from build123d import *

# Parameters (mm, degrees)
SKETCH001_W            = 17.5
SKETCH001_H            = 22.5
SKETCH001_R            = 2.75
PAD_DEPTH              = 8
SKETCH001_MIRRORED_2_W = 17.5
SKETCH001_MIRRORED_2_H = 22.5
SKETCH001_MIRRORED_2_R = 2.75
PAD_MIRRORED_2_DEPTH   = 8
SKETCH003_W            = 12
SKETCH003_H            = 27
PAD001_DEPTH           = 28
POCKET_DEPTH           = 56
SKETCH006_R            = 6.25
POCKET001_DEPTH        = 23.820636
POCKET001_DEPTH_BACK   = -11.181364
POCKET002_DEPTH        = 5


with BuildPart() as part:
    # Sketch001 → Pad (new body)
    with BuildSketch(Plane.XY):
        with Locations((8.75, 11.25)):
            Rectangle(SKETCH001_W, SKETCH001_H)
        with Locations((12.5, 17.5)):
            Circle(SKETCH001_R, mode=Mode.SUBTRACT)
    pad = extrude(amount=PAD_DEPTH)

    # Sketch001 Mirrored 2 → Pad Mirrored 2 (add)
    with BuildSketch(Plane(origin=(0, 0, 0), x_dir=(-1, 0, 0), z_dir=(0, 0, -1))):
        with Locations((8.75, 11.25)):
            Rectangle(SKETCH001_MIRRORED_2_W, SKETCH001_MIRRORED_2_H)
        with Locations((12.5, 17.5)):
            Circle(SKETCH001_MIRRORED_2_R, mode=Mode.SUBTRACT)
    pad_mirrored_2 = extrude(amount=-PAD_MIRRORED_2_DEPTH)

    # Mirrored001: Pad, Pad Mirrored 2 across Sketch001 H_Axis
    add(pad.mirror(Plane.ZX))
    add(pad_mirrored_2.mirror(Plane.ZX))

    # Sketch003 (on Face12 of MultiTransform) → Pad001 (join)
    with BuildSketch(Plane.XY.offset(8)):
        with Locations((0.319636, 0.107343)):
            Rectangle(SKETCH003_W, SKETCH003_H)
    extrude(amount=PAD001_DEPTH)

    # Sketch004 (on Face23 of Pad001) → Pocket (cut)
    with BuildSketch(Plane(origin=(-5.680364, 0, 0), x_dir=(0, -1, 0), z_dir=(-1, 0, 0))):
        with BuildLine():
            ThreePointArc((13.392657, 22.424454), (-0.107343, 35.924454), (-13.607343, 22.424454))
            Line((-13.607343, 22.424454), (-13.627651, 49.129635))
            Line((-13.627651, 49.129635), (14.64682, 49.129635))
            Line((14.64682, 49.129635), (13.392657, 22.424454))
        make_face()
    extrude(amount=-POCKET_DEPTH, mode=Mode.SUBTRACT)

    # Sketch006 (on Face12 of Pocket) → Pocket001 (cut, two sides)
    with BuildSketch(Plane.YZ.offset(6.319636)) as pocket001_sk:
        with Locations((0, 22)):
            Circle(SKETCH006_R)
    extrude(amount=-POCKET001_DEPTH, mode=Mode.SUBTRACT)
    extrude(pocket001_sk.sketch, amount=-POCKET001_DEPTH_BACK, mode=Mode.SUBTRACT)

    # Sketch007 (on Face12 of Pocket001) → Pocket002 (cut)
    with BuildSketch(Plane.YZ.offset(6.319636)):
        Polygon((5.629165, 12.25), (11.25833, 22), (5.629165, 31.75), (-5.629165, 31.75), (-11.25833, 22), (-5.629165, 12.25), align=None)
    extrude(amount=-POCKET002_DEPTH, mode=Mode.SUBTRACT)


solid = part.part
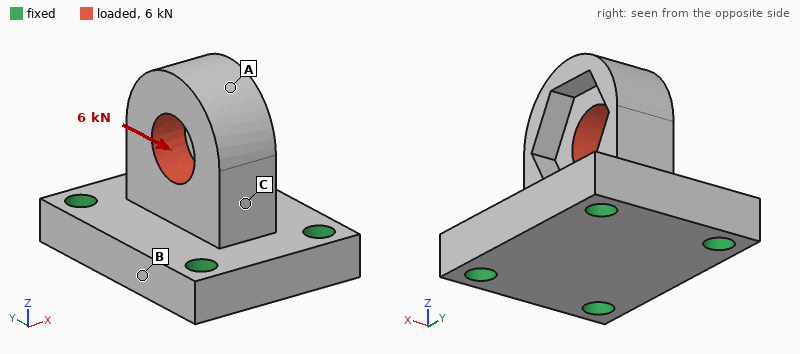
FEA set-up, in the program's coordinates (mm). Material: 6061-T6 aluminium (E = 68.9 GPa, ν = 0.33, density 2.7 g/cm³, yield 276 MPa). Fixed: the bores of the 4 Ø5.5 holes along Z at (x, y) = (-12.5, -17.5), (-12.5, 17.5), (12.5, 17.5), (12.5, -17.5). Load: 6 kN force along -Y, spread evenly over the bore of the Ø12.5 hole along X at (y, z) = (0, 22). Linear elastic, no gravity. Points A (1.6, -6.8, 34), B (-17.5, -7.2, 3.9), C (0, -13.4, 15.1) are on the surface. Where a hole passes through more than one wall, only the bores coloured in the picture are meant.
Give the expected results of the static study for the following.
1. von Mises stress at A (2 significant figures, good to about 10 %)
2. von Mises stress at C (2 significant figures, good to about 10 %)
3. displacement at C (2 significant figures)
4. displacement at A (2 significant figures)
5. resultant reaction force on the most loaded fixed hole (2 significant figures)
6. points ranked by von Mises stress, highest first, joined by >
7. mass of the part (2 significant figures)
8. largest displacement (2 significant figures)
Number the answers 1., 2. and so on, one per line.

1. 32 MPa
2. 84 MPa
3. 31 µm
4. 83 µm
5. 2.5 kN
6. C > A > B
7. 47 g
8. 85 µm
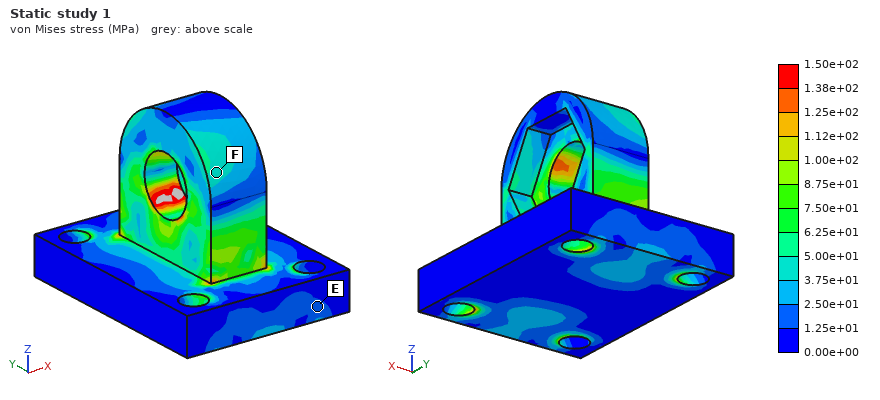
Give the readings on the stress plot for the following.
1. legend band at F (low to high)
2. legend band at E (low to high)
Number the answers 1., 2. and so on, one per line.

1. 3.75e+01 to 5.00e+01 MPa
2. 1.25e+01 to 2.50e+01 MPa
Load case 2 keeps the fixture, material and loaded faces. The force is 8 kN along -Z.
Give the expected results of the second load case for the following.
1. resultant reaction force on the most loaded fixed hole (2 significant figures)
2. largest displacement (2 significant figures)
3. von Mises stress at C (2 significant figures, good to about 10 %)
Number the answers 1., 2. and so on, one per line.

1. 2.5 kN
2. 53 µm
3. 38 MPa
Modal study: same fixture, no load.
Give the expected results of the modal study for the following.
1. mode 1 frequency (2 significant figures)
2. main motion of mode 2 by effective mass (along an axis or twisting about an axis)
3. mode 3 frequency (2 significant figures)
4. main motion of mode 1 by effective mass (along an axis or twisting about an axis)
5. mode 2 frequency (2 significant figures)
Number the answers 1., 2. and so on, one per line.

1. 9000 Hz
2. along Y
3. 19 kHz
4. along X
5. 13 kHz
